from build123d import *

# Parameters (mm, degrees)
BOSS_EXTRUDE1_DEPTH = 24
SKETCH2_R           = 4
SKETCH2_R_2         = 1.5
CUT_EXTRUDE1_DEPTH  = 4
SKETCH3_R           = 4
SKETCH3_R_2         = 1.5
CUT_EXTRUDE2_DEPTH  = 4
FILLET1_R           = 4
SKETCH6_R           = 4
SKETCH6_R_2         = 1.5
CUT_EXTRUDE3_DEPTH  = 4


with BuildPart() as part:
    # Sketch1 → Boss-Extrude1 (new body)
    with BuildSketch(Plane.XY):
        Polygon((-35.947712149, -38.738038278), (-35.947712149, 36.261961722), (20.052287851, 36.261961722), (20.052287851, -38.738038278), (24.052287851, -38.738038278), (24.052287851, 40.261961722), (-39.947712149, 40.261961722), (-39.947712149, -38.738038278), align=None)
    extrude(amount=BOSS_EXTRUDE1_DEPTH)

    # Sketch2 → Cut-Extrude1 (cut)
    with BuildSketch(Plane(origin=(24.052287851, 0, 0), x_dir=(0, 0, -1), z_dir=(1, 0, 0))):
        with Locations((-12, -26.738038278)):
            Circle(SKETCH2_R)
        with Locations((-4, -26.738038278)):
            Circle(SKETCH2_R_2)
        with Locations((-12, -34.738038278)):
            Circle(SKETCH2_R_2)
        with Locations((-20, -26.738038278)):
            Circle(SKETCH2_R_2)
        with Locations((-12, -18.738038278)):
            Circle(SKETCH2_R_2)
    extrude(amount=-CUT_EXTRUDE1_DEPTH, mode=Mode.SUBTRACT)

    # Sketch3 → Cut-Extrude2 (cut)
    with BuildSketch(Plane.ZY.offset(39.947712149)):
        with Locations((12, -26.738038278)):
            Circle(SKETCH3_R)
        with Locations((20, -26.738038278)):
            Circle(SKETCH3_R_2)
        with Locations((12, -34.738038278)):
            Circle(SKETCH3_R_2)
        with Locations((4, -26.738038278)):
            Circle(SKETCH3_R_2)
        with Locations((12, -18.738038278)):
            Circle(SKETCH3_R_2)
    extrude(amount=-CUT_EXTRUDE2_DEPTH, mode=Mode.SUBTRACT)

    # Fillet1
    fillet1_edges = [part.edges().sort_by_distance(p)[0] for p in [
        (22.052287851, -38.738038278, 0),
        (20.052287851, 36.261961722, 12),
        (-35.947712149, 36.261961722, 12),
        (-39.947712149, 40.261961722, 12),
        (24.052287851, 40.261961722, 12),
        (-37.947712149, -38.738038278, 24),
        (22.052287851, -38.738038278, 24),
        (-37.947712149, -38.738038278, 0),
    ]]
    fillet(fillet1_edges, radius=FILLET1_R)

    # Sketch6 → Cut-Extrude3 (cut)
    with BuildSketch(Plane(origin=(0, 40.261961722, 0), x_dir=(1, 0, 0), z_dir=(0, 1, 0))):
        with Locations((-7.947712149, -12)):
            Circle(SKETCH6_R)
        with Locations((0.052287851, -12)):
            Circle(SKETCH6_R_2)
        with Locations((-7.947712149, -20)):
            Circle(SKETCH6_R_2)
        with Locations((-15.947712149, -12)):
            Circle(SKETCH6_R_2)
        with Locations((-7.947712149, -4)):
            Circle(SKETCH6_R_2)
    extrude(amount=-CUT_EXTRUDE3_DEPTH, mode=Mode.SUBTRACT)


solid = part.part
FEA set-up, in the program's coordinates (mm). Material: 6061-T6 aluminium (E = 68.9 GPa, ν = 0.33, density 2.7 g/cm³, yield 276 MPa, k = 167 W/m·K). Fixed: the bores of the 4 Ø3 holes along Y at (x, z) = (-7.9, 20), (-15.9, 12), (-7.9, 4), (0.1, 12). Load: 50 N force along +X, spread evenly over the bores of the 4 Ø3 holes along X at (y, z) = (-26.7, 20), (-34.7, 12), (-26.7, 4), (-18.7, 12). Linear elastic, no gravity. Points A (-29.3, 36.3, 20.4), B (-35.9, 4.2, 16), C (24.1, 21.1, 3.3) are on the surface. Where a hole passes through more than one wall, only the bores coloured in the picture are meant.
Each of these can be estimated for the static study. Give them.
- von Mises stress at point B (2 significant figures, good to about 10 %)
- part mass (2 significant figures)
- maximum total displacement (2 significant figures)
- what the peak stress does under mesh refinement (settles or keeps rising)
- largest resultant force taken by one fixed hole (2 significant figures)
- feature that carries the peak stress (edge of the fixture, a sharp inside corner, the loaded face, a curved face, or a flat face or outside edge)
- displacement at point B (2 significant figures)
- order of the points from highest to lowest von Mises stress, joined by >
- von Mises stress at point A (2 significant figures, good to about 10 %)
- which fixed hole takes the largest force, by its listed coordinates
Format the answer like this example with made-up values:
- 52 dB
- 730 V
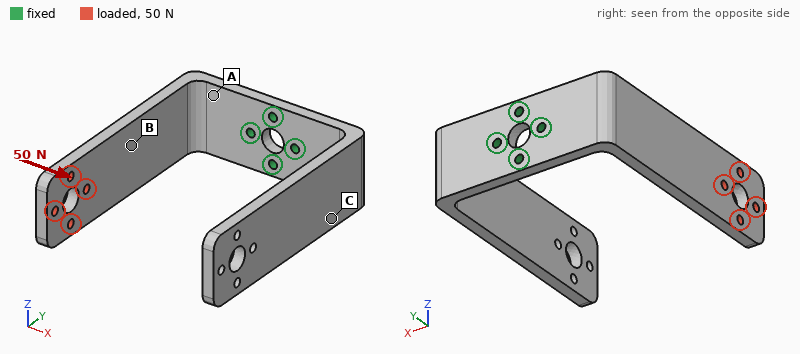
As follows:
- 24 MPa
- 53 g
- 1.1 mm
- keeps rising
- 210 N
- edge of the fixture
- 0.39 mm
- A > B > C
- 48 MPa
- (-15.9, 12)
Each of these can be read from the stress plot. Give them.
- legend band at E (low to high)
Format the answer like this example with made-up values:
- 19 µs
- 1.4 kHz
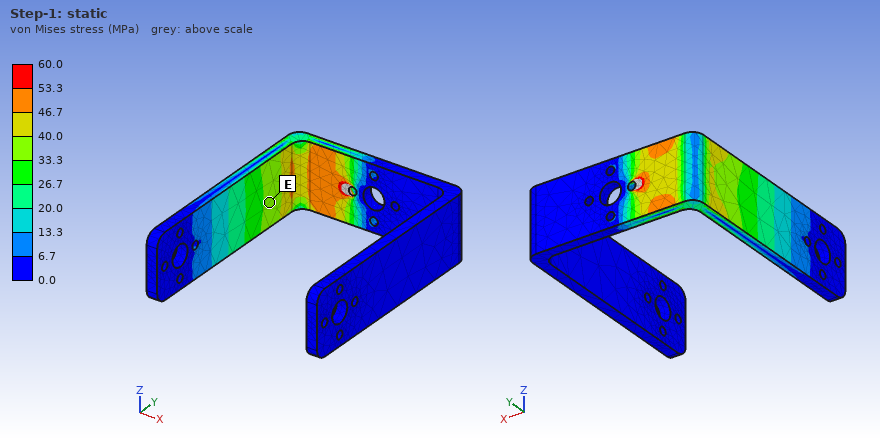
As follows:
- 33.3 to 40.0 MPa
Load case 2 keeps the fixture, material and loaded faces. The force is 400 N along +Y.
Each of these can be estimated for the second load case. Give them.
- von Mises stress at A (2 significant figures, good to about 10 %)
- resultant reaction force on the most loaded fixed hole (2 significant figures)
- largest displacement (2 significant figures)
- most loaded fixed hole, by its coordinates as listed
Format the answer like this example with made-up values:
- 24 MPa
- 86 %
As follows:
- 52 MPa
- 820 N
- 0.88 mm
- (-15.9, 12)
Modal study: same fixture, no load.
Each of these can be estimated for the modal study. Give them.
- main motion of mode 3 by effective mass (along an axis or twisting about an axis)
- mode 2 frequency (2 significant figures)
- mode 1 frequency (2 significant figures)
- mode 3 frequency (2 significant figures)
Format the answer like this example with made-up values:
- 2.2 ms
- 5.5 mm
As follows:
- twisting about Y
- 420 Hz
- 420 Hz
- 680 Hz
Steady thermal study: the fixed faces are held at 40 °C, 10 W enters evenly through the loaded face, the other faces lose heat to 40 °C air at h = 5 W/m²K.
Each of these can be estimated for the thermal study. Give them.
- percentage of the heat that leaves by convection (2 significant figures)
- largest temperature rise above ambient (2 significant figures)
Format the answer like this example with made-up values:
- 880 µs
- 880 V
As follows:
- 7.8 %
- 54 K
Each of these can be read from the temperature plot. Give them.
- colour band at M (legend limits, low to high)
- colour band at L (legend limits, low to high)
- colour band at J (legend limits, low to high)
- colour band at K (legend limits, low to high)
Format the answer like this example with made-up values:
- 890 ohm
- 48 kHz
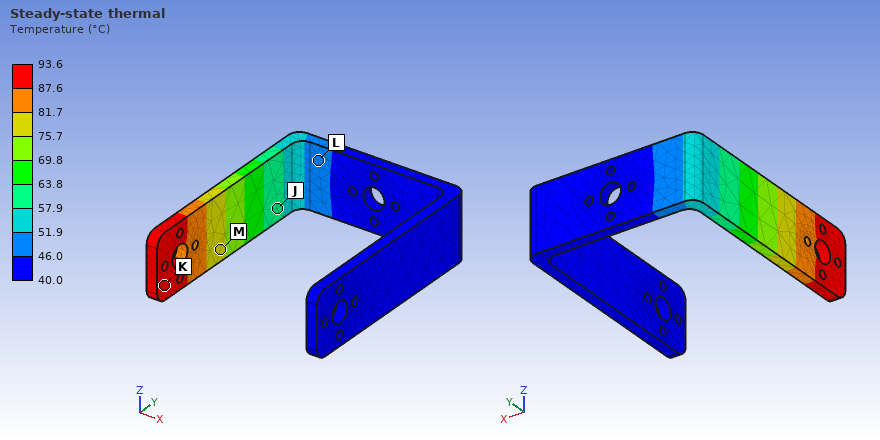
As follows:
- 75.7 to 81.7 °C
- 46.0 to 51.9 °C
- 57.9 to 63.8 °C
- 87.6 to 93.6 °C
